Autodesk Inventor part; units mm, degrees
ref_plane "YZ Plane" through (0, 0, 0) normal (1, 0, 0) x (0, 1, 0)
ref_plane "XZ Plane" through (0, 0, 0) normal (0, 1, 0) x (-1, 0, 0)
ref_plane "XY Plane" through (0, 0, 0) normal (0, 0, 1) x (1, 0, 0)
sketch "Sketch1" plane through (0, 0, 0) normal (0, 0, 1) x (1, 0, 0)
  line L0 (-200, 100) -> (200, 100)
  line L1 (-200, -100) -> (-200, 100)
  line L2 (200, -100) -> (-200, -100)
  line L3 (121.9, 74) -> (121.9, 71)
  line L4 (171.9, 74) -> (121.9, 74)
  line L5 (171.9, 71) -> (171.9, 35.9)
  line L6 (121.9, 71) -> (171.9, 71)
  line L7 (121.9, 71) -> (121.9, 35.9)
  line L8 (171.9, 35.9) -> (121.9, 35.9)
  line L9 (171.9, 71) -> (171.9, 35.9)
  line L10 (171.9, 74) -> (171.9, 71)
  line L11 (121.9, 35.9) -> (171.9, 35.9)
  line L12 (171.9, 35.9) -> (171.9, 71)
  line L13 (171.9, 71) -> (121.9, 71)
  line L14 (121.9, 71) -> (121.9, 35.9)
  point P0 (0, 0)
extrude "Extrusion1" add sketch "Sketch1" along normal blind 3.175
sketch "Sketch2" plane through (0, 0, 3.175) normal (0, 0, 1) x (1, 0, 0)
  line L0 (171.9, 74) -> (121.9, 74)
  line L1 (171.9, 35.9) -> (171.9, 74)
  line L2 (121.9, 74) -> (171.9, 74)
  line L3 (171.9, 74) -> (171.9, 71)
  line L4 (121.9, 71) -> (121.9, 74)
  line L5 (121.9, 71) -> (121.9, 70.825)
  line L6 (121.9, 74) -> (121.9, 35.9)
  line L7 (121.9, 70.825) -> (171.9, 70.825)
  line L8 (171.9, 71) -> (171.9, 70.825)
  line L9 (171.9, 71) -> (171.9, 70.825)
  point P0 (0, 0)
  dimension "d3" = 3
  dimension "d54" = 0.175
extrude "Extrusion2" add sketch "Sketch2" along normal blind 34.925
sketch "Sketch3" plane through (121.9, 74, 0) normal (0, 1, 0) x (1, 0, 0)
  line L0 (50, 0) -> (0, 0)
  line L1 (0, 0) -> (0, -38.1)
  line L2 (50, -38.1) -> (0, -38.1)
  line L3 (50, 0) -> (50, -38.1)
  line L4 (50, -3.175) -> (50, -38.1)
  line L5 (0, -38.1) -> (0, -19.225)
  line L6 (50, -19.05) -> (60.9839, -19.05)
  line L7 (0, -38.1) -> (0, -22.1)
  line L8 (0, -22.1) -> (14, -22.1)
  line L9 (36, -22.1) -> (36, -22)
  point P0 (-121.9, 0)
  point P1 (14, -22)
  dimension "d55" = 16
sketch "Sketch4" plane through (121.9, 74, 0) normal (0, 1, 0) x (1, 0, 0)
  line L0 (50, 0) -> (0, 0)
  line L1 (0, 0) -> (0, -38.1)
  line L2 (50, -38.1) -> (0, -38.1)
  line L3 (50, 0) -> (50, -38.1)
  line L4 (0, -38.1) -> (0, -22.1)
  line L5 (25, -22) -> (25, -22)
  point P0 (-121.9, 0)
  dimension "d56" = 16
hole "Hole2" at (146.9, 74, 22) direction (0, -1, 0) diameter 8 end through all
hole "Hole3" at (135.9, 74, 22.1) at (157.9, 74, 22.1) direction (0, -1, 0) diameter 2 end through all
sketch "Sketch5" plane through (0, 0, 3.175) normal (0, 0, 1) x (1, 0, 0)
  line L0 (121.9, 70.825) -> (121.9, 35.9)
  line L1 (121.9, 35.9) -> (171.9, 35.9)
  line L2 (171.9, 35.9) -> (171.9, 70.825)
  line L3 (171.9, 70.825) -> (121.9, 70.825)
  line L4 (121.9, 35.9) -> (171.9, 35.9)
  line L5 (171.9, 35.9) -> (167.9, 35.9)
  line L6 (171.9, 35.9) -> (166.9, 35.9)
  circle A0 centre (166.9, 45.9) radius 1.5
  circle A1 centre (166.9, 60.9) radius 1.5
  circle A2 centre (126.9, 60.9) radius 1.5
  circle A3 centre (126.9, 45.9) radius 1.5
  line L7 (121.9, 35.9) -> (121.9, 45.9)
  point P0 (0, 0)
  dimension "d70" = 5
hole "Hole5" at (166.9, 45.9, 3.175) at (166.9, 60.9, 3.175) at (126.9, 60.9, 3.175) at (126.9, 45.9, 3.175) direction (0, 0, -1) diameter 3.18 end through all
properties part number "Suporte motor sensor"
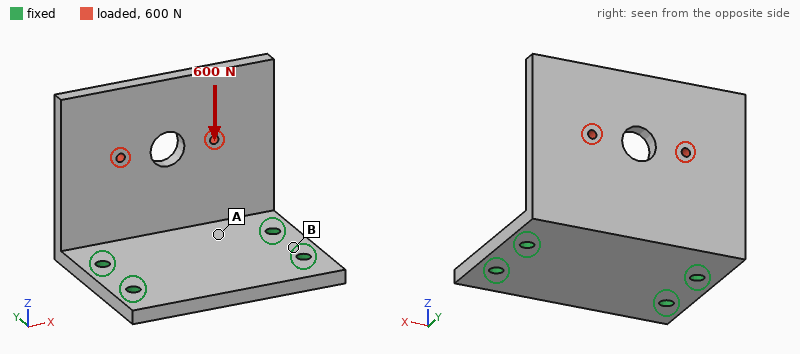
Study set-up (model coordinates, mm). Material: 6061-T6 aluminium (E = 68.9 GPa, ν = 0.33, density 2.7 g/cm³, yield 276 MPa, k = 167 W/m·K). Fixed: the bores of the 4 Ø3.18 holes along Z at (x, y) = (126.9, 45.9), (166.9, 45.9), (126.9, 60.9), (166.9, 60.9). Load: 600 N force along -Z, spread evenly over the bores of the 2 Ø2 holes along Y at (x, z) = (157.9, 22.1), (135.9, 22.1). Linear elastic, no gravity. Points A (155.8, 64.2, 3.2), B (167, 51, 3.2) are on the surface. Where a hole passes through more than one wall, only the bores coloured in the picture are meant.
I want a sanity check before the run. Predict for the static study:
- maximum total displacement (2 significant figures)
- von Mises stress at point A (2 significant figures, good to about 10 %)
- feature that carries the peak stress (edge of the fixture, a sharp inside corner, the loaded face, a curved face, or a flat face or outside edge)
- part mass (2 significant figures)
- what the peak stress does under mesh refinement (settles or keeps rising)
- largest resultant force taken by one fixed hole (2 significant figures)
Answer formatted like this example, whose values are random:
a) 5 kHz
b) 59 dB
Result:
a) 0.19 mm
b) 32 MPa
c) edge of the fixture
d) 31 g
e) keeps rising
f) 370 N
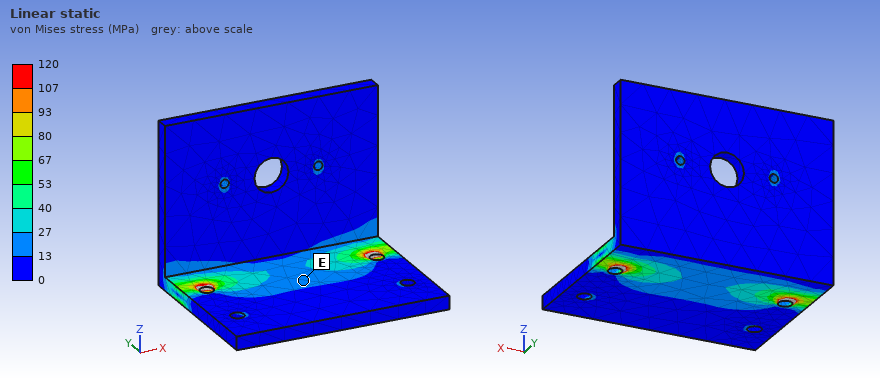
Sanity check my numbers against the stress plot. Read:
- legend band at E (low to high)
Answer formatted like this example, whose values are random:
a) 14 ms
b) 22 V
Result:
a) 13 to 27 MPa
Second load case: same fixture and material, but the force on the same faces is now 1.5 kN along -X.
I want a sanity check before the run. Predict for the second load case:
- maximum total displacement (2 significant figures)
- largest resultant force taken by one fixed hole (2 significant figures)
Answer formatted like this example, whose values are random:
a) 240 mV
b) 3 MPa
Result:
a) 0.24 mm
b) 1.1 kN
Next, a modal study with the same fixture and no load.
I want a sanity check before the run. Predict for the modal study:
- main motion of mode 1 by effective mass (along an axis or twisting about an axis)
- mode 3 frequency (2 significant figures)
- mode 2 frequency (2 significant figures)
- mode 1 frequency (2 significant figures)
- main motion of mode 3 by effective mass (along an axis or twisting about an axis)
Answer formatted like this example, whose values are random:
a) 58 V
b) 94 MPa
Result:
a) along Y
b) 4800 Hz
c) 3000 Hz
d) 1300 Hz
e) along X
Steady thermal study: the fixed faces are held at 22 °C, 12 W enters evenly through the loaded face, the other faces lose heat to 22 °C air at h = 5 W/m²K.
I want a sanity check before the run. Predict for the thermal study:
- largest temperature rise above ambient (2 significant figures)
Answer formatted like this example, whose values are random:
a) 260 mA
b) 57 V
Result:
a) 19 K
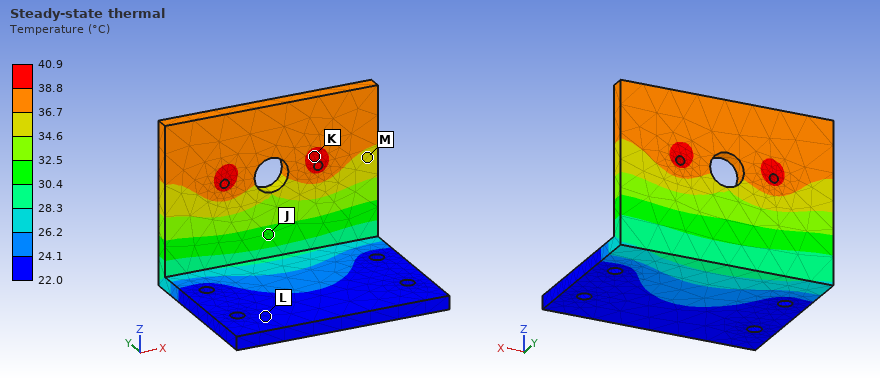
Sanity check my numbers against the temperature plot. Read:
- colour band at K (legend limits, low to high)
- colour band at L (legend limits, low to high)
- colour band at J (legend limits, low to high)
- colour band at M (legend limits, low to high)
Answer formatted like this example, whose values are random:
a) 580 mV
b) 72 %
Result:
a) 38.8 to 40.9 °C
b) 22.0 to 24.1 °C
c) 30.4 to 32.5 °C
d) 34.6 to 36.7 °C
